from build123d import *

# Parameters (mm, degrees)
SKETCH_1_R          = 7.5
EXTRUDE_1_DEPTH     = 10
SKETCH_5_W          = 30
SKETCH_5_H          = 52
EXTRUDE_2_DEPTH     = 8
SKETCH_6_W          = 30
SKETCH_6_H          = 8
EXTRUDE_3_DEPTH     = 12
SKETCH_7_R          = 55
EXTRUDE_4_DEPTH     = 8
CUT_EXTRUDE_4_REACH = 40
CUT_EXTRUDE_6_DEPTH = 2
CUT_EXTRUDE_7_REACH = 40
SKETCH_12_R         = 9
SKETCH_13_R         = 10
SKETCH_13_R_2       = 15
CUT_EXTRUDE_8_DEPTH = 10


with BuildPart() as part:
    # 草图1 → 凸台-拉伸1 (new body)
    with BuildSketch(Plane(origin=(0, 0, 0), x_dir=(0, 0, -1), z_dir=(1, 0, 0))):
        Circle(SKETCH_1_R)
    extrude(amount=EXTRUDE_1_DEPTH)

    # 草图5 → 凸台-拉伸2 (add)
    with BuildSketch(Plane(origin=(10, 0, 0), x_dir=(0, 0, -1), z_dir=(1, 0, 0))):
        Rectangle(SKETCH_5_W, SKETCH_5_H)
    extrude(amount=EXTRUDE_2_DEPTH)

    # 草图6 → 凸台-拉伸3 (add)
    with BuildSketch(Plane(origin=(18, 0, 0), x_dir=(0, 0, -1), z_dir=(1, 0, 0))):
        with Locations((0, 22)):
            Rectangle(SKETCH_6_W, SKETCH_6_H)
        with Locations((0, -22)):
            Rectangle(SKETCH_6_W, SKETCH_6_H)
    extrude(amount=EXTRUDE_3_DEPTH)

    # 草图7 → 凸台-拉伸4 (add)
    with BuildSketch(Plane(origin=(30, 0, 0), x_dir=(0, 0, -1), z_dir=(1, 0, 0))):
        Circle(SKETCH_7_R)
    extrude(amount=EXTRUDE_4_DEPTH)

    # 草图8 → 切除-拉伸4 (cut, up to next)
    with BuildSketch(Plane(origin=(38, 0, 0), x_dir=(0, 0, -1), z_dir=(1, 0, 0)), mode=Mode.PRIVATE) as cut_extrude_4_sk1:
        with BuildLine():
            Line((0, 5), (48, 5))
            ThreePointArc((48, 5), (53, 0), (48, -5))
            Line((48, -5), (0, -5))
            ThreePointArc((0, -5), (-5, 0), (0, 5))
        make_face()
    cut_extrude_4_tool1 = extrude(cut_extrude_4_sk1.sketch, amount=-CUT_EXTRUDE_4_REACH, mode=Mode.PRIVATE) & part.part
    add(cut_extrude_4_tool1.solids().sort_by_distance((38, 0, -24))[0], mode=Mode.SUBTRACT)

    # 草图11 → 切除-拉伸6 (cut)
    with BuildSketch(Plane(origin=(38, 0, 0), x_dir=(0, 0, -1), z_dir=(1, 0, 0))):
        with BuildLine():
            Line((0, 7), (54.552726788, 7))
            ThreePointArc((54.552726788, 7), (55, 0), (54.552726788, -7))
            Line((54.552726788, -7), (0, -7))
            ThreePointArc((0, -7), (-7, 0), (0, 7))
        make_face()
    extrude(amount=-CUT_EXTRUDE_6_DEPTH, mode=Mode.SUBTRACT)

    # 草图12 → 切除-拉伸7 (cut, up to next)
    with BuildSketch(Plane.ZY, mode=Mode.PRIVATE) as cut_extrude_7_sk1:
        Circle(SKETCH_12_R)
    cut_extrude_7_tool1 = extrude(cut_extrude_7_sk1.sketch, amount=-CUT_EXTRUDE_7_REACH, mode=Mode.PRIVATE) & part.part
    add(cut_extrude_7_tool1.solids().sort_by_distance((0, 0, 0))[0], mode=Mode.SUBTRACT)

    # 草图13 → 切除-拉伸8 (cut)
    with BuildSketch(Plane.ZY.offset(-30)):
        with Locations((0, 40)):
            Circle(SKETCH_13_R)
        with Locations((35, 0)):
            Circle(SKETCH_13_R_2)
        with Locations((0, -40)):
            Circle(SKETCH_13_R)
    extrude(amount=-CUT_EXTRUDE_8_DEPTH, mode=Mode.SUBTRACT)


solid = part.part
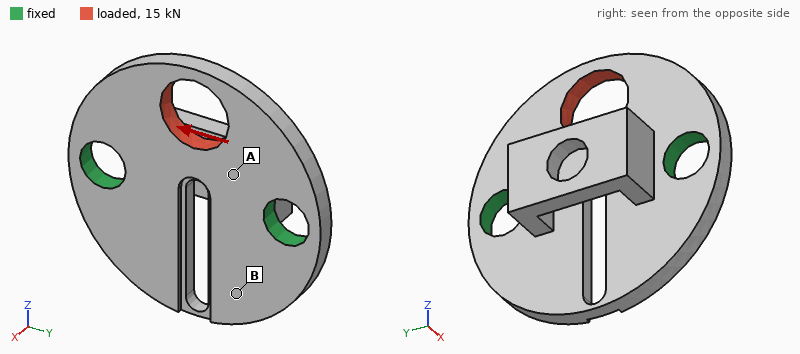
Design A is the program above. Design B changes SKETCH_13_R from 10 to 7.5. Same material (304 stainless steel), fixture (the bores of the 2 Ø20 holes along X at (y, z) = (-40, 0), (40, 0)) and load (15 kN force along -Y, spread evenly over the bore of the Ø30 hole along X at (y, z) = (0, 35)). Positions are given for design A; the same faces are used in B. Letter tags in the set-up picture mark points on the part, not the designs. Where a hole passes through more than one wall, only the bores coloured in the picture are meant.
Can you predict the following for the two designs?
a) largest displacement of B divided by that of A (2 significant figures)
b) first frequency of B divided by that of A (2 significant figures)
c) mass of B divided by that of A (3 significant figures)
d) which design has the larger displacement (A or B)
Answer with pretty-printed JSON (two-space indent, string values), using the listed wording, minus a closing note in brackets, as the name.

{
  "largest displacement of B divided by that of A": "1.1",
  "first frequency of B divided by that of A": "0.87",
  "mass of B divided by that of A": "1.03",
  "which design has the larger displacement": "B"
}
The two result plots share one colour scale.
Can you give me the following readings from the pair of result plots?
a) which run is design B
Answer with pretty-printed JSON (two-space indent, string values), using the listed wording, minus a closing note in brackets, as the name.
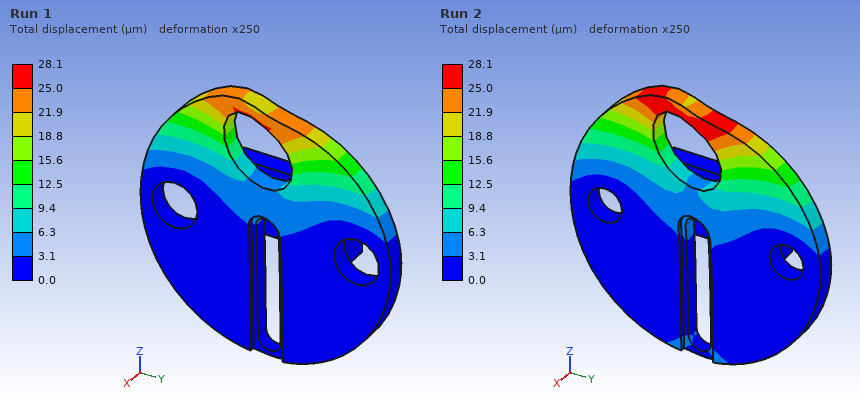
{
  "which run is design B": "Run 2"
}
